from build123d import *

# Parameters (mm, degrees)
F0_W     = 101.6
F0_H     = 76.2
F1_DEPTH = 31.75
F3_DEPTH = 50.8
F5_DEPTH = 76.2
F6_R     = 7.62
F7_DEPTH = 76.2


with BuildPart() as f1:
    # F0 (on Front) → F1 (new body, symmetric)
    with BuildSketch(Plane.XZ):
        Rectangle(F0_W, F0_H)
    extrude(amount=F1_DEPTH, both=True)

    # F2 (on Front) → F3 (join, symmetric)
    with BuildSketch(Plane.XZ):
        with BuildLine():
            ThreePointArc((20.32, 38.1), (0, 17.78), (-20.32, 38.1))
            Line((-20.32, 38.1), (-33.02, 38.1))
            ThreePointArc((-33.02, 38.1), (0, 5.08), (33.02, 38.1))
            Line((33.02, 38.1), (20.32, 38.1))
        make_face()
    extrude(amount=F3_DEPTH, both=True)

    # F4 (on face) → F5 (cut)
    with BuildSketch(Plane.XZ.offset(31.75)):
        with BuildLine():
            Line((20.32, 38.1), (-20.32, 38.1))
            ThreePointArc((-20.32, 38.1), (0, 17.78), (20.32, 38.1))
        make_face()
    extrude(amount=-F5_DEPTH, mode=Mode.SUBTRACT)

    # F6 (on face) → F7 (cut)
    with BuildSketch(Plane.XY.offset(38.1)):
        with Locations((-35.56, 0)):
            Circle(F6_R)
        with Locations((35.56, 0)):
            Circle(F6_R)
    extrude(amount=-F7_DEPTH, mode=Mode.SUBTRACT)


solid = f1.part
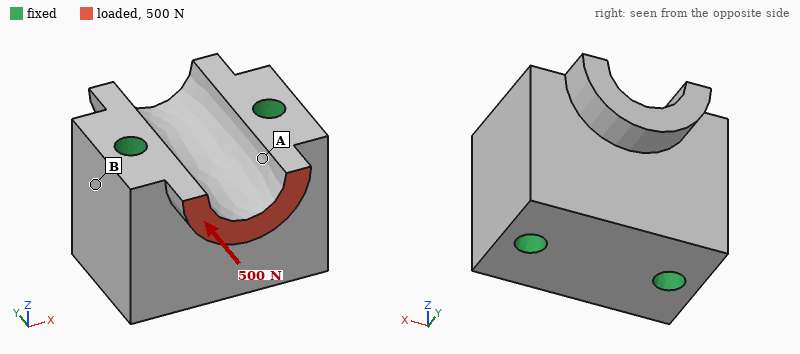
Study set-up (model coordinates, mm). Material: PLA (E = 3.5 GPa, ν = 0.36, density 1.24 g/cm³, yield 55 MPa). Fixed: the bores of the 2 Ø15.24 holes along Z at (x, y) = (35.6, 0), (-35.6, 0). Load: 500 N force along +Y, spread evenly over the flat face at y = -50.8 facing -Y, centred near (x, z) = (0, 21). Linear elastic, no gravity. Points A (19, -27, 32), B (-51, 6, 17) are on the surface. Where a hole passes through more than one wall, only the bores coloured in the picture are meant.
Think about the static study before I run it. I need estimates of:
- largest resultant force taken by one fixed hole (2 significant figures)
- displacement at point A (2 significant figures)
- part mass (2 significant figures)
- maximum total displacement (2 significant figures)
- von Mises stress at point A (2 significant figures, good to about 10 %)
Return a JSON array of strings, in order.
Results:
["260 N", "3.4 µm", "570 g", "7.5 µm", "0.40 MPa"]
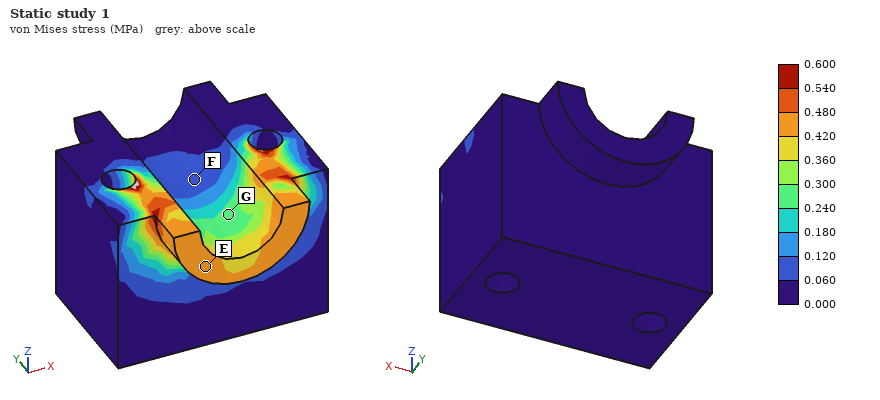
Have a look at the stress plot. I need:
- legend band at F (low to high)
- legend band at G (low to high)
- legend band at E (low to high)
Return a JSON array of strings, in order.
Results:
["0.060 to 0.120 MPa", "0.240 to 0.300 MPa", "0.420 to 0.480 MPa"]
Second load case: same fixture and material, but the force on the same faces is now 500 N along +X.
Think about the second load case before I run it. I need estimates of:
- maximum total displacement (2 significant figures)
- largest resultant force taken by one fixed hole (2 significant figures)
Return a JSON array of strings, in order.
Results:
["45 µm", "390 N"]
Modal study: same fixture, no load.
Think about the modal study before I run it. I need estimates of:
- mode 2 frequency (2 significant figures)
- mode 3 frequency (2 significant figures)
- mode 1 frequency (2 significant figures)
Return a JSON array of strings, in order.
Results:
["4800 Hz", "4900 Hz", "4800 Hz"]
